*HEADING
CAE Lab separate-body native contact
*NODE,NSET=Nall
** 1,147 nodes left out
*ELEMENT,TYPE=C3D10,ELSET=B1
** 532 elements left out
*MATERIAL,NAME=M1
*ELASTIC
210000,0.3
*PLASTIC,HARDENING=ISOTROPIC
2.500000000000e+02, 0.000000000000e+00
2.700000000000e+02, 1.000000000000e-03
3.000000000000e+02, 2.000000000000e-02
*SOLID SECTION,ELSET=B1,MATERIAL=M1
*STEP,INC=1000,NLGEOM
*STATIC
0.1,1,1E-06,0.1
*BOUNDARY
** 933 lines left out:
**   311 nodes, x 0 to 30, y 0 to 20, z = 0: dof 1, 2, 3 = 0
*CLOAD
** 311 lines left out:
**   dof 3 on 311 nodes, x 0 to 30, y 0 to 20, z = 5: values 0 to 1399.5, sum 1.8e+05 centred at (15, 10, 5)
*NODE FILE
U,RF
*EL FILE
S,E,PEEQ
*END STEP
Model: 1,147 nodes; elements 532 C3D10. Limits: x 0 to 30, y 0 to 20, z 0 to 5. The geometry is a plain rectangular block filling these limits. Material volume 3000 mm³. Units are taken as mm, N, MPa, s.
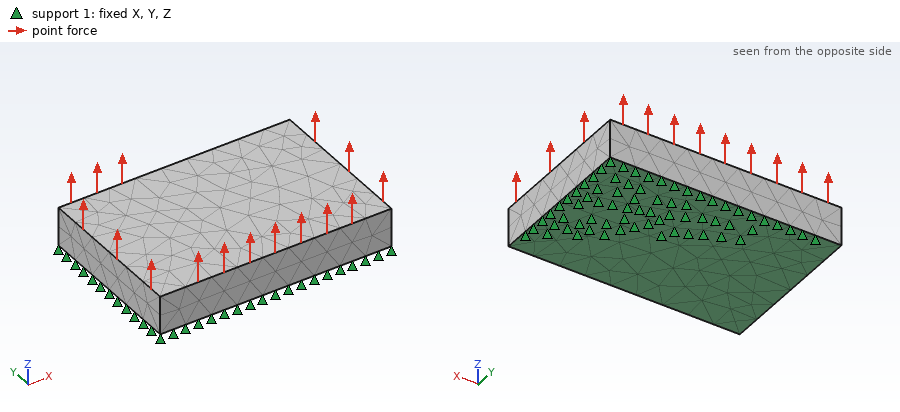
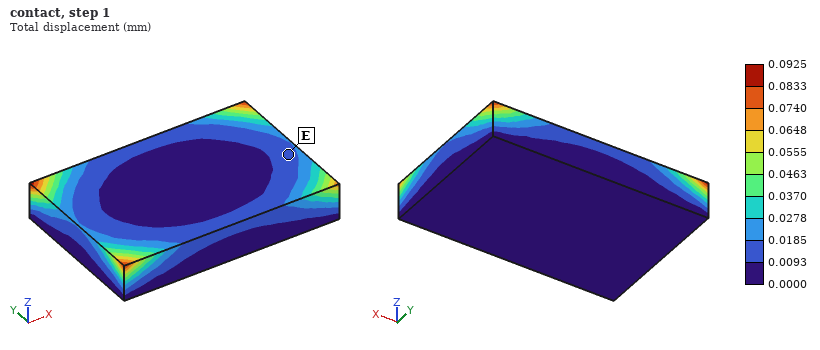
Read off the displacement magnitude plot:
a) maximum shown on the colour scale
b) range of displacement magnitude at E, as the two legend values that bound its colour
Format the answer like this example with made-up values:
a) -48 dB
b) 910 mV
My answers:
a) 0.0925 mm
b) 0.0093 to 0.0185 mm
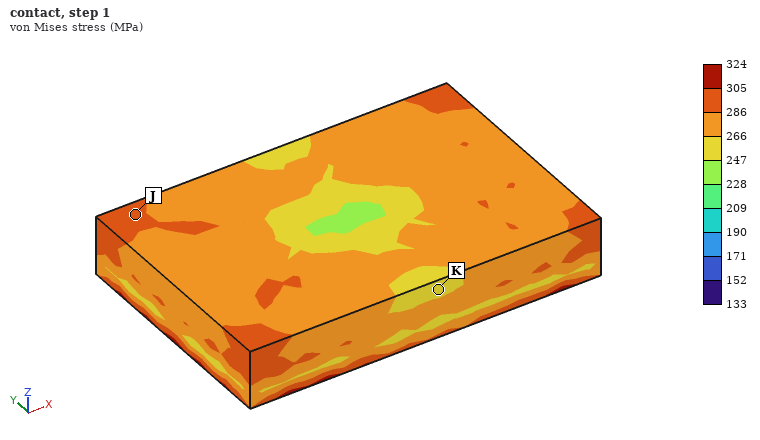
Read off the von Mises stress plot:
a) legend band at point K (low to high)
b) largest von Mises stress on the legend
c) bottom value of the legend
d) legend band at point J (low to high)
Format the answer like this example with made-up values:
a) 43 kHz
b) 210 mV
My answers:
a) 247 to 266 MPa
b) 324 MPa
c) 133 MPa
d) 286 to 305 MPa
